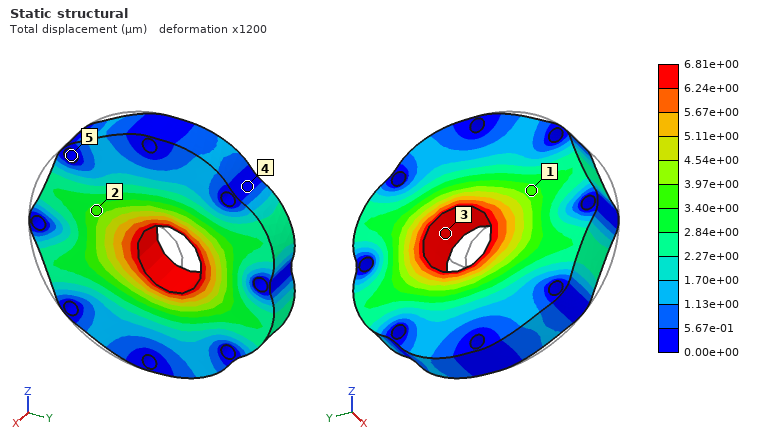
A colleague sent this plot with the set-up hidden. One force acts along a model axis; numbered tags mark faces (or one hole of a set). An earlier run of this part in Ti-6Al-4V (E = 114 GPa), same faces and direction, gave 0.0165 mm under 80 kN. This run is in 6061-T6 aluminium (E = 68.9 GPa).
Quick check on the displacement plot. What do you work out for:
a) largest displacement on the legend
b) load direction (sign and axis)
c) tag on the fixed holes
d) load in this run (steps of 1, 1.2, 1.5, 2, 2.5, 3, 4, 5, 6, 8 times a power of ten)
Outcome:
6.81e+00 µm
+Y
5
20 kN
